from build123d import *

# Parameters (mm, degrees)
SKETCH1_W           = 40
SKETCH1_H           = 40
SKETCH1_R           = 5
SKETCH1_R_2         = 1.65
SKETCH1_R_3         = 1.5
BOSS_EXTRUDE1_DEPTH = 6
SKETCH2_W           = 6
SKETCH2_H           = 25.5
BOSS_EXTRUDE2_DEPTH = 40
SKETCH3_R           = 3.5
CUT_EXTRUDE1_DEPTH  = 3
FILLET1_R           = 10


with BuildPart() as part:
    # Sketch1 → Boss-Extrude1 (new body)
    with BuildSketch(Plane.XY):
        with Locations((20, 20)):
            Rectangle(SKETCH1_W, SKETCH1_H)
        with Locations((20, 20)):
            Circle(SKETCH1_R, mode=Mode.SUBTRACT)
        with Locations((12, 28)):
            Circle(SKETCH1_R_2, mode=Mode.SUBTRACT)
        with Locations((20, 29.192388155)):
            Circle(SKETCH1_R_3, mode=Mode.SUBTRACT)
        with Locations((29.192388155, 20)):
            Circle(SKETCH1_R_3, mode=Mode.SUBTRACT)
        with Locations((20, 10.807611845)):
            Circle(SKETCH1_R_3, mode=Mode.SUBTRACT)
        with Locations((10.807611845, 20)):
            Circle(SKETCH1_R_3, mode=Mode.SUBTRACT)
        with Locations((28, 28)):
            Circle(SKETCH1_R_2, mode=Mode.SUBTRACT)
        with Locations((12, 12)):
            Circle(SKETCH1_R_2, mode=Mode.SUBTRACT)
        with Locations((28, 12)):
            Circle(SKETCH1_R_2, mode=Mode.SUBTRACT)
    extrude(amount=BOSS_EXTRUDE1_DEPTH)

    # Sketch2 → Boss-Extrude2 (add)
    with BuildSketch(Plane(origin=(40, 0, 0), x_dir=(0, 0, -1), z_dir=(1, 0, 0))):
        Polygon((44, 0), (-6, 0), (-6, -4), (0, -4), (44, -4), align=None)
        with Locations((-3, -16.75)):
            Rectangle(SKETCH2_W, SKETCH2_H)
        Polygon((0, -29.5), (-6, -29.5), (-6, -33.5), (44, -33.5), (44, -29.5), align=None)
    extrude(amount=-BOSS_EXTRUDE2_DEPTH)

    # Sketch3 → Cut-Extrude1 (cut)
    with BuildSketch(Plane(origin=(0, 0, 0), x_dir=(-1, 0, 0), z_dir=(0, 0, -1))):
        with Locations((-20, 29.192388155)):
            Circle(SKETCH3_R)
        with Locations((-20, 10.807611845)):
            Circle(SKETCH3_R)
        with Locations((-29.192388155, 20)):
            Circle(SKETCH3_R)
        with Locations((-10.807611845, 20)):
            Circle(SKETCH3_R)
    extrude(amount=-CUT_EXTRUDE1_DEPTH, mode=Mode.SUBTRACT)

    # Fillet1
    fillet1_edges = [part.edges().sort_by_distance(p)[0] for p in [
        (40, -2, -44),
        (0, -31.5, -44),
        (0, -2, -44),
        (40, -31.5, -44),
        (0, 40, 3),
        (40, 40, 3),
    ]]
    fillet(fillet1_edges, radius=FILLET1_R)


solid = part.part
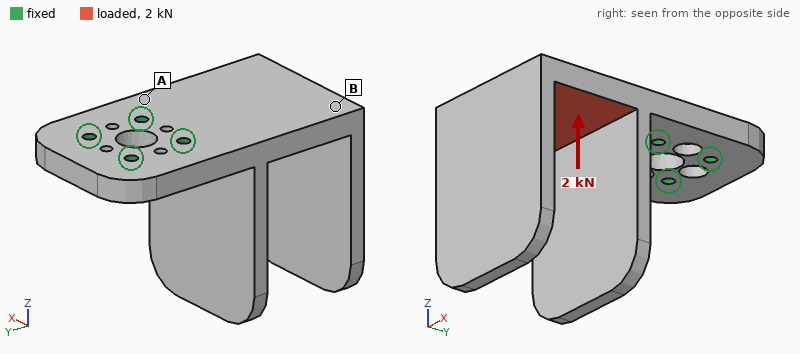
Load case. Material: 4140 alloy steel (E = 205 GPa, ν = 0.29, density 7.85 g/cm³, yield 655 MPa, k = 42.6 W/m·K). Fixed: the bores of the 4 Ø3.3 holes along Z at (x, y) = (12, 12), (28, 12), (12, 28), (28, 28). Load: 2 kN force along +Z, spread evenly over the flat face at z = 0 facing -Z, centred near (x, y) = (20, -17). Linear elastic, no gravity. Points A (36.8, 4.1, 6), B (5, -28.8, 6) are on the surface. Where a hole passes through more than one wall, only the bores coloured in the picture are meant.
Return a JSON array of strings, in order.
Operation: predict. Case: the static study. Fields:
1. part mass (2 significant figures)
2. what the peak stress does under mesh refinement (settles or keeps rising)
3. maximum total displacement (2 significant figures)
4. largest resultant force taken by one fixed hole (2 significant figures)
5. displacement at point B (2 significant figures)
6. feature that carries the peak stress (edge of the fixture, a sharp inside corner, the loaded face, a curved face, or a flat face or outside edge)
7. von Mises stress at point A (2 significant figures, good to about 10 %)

["230 g", "keeps rising", "0.37 mm", "1.5 kN", "0.20 mm", "edge of the fixture", "160 MPa"]
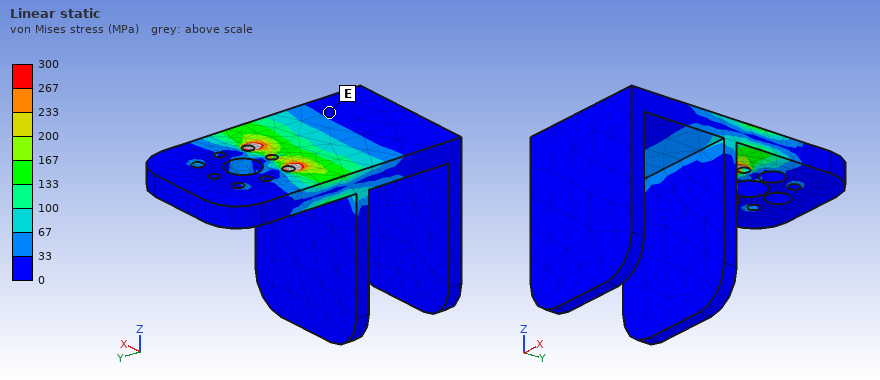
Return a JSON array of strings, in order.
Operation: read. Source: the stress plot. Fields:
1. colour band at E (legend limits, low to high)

["0 to 33 MPa"]
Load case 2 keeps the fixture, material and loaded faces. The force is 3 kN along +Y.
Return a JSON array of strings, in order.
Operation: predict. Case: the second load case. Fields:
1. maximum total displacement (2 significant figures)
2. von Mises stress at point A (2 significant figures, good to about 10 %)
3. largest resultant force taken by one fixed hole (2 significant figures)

["98 µm", "25 MPa", "1.3 kN"]
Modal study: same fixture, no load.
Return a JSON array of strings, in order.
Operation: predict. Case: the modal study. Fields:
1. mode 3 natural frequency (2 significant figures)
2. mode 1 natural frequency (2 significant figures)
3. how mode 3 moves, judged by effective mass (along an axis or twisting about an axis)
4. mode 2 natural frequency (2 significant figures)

["1700 Hz", "880 Hz", "along X", "1500 Hz"]
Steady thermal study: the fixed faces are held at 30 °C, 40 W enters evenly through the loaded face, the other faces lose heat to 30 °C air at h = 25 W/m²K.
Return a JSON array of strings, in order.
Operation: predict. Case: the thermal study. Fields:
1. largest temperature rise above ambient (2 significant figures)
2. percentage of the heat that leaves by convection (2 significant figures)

["80 K", "34 %"]
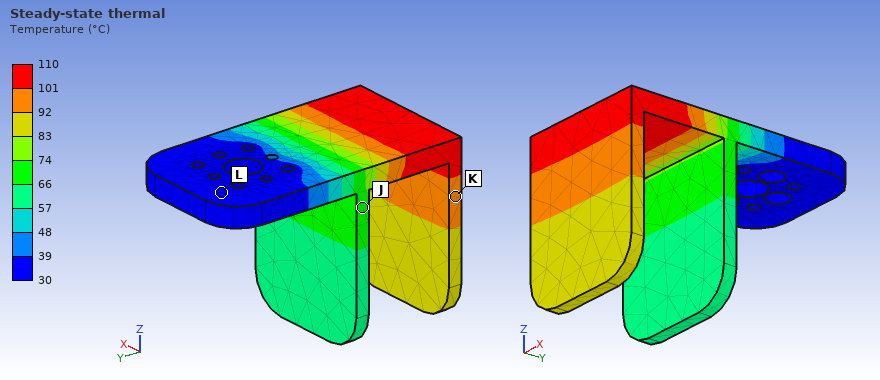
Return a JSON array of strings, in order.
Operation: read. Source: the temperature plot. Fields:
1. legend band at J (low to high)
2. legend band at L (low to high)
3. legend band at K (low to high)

["66 to 74 °C", "30 to 39 °C", "92 to 101 °C"]
